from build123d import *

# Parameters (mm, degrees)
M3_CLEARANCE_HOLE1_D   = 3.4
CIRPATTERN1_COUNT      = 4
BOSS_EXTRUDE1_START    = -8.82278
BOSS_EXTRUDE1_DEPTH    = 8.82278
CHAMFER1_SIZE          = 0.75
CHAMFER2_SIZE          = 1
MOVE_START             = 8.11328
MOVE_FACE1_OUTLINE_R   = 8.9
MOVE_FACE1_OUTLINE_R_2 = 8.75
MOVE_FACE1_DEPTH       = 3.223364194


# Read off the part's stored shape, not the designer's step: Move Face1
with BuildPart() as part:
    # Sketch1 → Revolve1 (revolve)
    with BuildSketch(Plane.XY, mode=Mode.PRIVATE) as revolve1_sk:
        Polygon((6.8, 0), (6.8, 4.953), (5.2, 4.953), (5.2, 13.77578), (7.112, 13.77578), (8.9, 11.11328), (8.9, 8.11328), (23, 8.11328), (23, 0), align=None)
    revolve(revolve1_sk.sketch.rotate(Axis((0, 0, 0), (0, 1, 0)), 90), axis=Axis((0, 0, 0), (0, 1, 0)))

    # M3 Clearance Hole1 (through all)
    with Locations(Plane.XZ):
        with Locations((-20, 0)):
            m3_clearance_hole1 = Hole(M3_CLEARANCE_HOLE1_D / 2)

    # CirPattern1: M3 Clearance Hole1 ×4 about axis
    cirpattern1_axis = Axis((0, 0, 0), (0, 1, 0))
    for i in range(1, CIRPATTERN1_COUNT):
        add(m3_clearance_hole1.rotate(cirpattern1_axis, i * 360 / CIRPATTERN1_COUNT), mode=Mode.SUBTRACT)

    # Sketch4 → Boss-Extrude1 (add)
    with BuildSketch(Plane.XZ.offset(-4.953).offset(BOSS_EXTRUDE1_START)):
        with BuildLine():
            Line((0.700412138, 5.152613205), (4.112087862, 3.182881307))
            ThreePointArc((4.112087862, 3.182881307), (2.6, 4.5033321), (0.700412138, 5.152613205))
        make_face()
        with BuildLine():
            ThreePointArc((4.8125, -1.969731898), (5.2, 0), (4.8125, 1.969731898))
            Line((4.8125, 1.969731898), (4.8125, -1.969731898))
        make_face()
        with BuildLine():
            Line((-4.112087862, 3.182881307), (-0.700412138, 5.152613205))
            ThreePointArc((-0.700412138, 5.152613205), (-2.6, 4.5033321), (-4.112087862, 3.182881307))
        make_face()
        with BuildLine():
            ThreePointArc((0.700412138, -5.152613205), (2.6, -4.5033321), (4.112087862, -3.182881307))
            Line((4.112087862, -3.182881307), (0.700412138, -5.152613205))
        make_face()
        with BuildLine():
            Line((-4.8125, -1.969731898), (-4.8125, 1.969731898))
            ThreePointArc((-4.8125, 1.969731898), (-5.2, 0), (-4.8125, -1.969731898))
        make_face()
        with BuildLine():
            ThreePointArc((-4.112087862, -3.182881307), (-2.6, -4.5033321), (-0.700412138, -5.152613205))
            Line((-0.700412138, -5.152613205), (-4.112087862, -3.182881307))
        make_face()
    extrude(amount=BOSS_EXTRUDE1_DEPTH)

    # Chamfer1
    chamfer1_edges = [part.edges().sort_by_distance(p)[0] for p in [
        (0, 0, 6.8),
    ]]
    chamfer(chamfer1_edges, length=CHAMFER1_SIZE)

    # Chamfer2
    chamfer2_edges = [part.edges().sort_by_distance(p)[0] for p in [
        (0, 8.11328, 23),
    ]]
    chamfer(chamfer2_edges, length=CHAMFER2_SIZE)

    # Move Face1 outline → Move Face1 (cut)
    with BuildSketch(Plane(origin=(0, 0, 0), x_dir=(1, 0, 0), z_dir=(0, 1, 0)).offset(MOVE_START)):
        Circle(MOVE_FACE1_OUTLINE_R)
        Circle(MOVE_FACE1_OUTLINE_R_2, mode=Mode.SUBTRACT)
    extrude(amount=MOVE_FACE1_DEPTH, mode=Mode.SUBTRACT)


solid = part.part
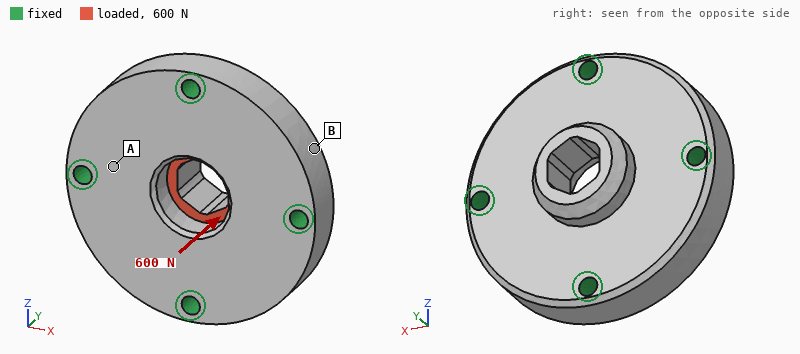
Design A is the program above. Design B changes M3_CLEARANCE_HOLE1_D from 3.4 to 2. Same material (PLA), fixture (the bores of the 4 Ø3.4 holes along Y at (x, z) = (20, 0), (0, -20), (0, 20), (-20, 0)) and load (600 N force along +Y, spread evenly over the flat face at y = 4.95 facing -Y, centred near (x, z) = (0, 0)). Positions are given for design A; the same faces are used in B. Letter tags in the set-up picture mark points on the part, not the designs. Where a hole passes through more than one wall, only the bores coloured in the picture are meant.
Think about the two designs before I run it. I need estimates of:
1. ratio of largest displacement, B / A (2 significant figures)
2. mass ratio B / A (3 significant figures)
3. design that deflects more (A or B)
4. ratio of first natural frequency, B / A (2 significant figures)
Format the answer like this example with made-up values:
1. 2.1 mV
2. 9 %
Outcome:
1. 1.1
2. 1.01
3. B
4. 0.89
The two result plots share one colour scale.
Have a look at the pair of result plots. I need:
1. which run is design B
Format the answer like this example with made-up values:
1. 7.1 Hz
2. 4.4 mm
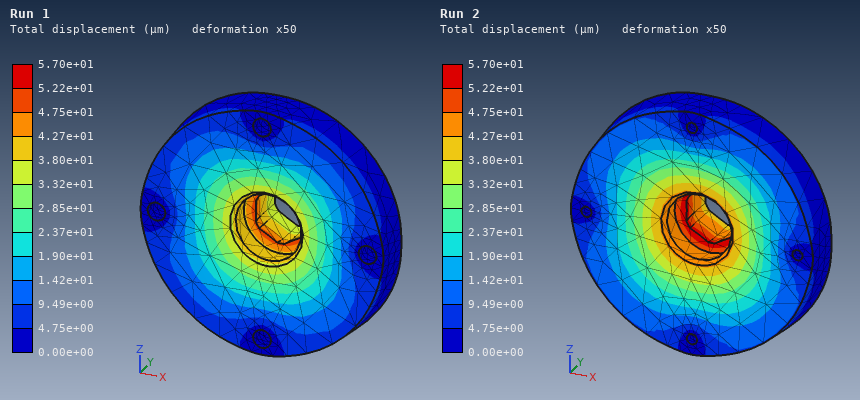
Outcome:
1. Run 2
